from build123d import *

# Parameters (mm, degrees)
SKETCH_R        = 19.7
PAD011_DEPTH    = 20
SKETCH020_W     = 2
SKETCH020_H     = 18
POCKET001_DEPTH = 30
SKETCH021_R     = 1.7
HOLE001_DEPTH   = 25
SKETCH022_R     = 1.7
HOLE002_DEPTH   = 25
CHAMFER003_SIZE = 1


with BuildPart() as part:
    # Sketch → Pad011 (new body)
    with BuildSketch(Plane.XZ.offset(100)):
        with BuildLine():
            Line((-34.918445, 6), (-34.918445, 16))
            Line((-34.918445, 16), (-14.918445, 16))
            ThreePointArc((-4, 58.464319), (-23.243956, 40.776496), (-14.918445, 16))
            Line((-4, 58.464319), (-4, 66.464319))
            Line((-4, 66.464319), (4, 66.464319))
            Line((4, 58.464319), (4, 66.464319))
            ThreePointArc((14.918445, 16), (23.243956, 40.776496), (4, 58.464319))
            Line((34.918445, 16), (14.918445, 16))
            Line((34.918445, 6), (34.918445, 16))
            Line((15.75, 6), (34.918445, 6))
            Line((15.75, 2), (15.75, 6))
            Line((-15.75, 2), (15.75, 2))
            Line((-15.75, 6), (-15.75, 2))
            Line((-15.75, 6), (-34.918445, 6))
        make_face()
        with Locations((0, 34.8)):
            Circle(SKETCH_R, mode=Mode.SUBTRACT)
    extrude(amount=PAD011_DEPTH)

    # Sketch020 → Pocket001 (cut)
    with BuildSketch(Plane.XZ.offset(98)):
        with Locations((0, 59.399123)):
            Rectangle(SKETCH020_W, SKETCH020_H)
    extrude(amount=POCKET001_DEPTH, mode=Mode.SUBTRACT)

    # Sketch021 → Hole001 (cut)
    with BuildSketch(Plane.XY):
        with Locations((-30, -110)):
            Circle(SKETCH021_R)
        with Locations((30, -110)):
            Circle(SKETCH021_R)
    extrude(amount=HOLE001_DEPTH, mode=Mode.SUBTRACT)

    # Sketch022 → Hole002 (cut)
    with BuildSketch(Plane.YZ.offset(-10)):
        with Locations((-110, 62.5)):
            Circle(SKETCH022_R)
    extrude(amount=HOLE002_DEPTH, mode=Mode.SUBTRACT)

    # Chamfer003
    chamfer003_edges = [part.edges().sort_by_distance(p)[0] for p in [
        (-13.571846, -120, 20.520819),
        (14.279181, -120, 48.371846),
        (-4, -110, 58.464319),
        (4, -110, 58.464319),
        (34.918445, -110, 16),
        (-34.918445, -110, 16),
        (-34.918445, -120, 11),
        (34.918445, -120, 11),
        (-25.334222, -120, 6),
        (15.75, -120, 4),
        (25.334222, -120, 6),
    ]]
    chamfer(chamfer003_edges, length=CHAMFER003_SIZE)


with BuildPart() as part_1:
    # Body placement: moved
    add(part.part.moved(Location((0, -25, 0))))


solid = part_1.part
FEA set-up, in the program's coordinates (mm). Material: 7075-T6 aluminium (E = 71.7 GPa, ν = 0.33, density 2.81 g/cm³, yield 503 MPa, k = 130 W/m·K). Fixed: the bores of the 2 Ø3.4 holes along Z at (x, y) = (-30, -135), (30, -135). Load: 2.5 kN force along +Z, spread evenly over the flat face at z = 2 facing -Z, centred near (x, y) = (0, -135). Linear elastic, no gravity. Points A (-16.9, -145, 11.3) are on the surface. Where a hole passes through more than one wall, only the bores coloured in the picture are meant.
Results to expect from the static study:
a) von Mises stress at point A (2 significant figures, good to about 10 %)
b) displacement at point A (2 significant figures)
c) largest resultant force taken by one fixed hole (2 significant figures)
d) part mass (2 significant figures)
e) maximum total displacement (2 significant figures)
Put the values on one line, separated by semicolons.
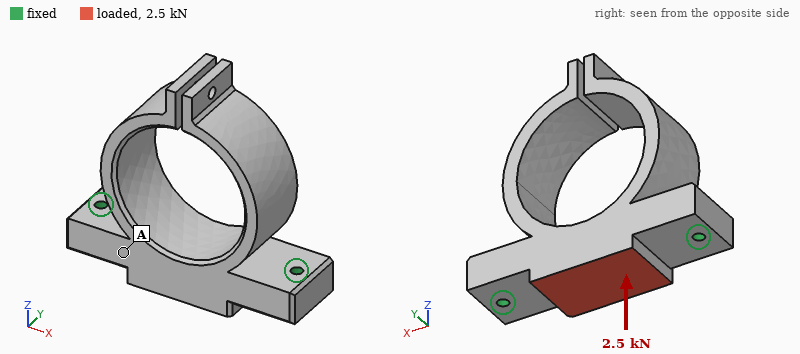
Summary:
13 MPa; 12 µm; 1.3 kN; 75 g; 37 µm
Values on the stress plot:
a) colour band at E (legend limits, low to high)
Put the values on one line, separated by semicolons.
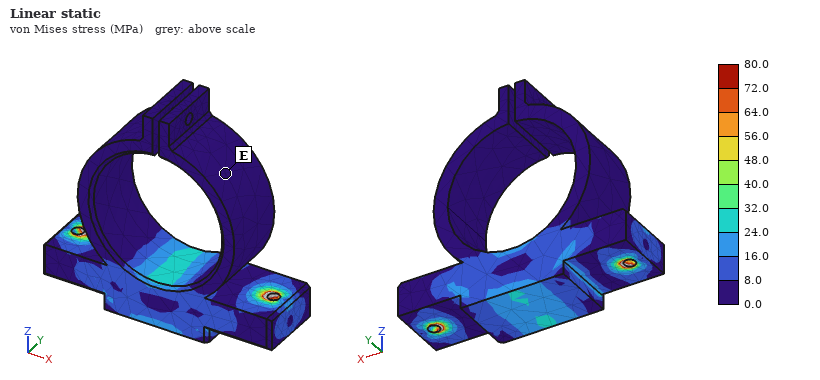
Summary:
0.0 to 8.0 MPa
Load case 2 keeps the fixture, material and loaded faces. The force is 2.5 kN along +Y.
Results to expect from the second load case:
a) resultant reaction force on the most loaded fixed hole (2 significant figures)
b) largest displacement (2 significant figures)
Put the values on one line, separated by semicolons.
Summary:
1.3 kN; 64 µm
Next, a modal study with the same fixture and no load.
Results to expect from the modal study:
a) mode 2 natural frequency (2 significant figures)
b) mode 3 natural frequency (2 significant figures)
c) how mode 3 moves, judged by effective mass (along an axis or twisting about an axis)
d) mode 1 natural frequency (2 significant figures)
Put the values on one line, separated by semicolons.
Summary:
1100 Hz; 1700 Hz; along Y; 1100 Hz
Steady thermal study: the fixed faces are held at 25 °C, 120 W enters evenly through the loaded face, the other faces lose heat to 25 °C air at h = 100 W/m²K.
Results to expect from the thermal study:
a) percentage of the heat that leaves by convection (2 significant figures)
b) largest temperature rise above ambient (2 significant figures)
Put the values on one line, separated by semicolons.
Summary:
19 %; 52 K
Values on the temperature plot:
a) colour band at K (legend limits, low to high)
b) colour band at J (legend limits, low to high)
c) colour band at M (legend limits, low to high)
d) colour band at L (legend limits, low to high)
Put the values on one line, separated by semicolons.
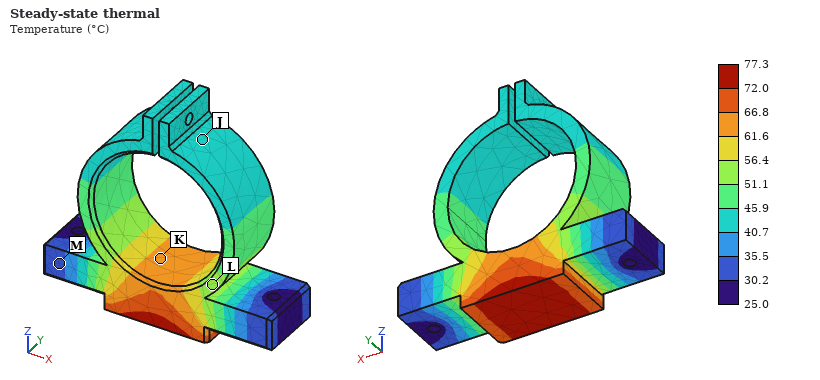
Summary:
61.6 to 66.8 °C; 40.7 to 45.9 °C; 30.2 to 35.5 °C; 51.1 to 56.4 °C
